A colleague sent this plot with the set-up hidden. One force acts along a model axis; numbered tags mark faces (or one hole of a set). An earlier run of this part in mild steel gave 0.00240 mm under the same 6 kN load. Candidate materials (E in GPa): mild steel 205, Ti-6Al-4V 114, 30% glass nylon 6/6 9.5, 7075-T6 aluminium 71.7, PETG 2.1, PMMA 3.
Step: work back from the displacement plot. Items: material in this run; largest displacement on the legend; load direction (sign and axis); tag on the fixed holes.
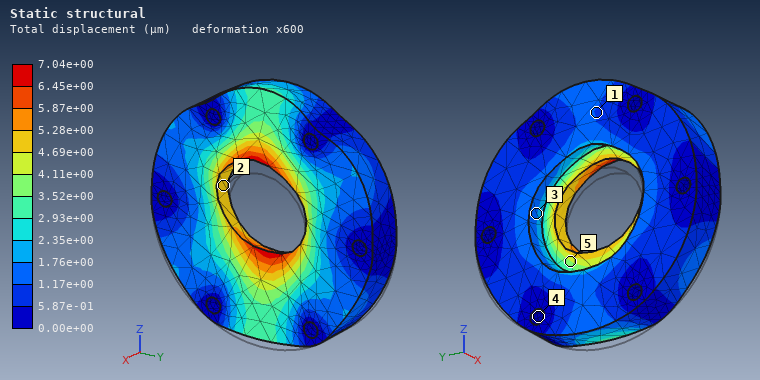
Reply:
7075-T6 aluminium
7.04e+00 µm
+Z
4
